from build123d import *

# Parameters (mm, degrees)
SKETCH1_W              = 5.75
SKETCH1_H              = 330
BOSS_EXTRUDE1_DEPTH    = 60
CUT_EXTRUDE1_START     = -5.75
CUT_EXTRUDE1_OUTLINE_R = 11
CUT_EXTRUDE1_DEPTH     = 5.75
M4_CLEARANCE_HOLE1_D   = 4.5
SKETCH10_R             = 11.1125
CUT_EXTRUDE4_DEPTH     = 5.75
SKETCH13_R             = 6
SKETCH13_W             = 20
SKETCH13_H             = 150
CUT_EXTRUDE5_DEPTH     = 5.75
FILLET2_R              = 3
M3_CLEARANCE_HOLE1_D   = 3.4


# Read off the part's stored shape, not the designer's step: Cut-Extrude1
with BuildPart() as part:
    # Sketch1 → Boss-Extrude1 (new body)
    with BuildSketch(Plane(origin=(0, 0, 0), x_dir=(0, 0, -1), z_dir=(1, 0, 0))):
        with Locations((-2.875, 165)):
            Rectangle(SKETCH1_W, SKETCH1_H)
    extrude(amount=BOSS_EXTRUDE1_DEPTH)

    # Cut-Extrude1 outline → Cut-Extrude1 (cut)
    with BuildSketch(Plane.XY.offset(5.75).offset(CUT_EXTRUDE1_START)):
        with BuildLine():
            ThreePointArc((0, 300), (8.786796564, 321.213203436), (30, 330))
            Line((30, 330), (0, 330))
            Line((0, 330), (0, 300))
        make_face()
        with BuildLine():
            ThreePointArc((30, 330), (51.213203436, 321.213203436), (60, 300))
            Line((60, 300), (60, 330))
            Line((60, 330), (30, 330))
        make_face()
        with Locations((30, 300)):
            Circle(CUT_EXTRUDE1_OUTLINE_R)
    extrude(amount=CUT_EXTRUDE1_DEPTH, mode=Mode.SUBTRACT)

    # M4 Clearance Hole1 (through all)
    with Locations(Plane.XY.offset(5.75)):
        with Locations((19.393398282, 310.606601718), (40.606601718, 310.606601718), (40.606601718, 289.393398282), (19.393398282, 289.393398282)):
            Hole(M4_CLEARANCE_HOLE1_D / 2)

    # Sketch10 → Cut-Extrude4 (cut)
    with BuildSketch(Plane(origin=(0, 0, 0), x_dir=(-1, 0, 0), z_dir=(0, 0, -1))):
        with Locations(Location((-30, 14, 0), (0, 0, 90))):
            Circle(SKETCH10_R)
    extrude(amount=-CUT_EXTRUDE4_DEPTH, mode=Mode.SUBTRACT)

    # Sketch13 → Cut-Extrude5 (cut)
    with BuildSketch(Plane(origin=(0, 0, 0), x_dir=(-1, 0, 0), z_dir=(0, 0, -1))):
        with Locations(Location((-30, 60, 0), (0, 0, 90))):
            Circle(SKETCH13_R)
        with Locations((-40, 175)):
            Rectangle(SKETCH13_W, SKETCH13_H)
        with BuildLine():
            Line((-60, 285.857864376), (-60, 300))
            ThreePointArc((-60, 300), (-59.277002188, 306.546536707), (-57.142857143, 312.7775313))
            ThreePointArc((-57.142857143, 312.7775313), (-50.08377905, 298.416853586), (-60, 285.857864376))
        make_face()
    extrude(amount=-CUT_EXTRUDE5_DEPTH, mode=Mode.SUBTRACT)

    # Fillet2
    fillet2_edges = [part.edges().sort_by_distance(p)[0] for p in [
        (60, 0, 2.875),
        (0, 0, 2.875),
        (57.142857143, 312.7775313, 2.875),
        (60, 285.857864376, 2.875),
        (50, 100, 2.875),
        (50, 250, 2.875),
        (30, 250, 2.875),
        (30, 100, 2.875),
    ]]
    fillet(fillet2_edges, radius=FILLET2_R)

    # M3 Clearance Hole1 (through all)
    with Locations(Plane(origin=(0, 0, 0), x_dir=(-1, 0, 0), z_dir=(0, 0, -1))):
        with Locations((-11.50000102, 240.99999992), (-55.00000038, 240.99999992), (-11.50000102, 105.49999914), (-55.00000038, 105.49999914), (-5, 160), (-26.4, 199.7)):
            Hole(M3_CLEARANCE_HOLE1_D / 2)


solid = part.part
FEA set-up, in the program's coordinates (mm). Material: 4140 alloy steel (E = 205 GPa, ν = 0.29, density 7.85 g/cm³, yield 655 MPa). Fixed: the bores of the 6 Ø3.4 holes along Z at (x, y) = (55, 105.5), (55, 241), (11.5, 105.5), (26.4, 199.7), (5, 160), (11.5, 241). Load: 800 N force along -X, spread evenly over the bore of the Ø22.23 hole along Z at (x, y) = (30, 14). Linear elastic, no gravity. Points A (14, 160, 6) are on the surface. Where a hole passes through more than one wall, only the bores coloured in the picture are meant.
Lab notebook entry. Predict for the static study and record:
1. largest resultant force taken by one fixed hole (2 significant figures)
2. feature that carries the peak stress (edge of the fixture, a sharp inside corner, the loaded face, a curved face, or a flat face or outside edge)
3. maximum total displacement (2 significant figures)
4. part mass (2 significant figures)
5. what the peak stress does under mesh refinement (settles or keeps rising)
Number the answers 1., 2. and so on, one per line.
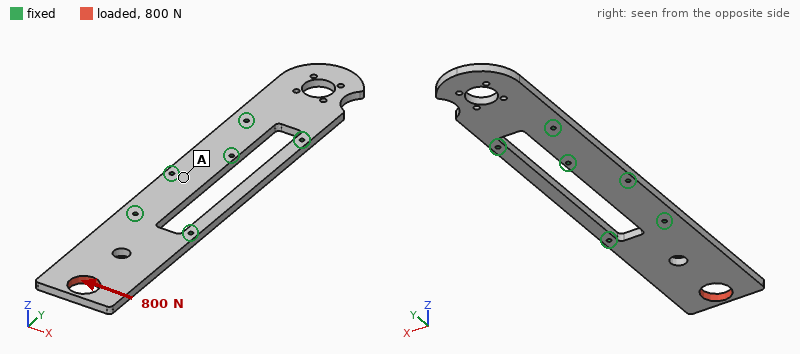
1. 1.6 kN
2. edge of the fixture
3. 20 µm
4. 690 g
5. keeps rising
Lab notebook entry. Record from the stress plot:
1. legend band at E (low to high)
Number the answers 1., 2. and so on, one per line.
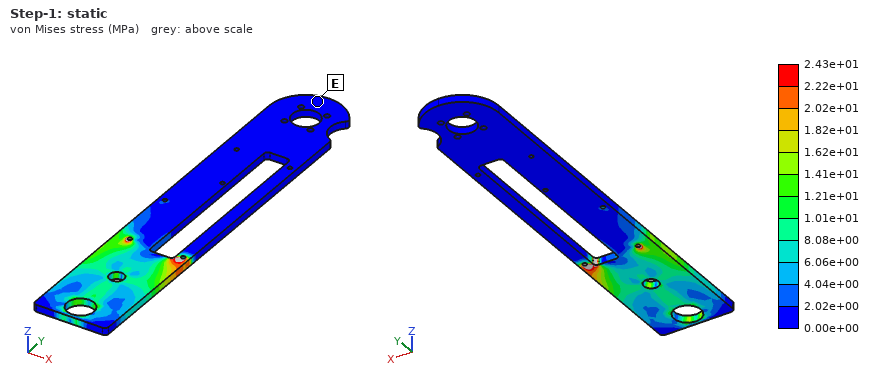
1. 0.00e+00 to 2.02e+00 MPa
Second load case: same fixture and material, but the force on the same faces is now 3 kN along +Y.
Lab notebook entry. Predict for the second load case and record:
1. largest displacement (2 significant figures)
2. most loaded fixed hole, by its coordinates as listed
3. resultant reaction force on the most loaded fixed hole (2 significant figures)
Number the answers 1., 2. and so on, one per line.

1. 10 µm
2. (11.5, 105.5)
3. 1.5 kN
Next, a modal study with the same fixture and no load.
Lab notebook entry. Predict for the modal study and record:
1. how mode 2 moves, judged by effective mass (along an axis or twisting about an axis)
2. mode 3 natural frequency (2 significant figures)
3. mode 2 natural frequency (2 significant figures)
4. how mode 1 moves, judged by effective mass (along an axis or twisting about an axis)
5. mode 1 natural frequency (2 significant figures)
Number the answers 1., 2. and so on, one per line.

1. along Z
2. 1500 Hz
3. 640 Hz
4. along Z
5. 410 Hz
